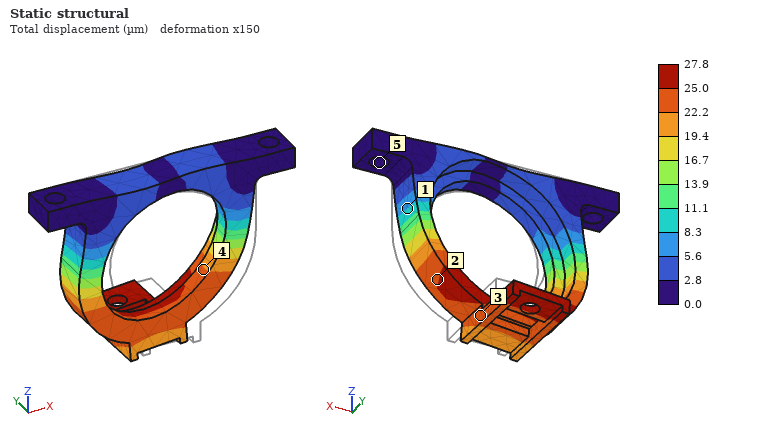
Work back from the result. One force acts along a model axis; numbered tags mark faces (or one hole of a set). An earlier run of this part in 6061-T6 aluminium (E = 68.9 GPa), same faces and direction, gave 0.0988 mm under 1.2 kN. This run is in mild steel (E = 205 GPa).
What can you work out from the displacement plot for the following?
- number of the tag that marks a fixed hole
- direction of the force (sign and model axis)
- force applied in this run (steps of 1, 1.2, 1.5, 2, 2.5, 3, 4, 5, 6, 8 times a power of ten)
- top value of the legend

5
-X
1 kN
27.8 µm
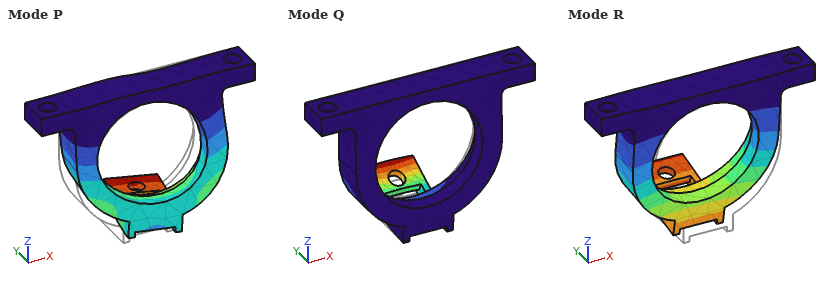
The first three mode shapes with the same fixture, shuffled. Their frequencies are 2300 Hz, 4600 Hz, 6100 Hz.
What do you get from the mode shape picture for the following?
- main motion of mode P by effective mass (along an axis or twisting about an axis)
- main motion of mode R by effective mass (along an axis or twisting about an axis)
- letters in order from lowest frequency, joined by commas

along X
along Y
R, P, Q
